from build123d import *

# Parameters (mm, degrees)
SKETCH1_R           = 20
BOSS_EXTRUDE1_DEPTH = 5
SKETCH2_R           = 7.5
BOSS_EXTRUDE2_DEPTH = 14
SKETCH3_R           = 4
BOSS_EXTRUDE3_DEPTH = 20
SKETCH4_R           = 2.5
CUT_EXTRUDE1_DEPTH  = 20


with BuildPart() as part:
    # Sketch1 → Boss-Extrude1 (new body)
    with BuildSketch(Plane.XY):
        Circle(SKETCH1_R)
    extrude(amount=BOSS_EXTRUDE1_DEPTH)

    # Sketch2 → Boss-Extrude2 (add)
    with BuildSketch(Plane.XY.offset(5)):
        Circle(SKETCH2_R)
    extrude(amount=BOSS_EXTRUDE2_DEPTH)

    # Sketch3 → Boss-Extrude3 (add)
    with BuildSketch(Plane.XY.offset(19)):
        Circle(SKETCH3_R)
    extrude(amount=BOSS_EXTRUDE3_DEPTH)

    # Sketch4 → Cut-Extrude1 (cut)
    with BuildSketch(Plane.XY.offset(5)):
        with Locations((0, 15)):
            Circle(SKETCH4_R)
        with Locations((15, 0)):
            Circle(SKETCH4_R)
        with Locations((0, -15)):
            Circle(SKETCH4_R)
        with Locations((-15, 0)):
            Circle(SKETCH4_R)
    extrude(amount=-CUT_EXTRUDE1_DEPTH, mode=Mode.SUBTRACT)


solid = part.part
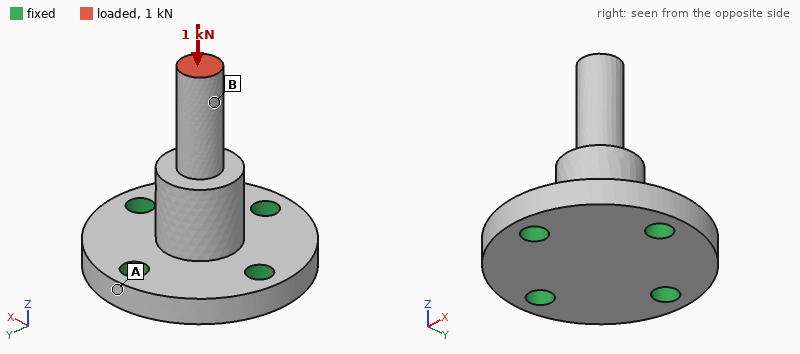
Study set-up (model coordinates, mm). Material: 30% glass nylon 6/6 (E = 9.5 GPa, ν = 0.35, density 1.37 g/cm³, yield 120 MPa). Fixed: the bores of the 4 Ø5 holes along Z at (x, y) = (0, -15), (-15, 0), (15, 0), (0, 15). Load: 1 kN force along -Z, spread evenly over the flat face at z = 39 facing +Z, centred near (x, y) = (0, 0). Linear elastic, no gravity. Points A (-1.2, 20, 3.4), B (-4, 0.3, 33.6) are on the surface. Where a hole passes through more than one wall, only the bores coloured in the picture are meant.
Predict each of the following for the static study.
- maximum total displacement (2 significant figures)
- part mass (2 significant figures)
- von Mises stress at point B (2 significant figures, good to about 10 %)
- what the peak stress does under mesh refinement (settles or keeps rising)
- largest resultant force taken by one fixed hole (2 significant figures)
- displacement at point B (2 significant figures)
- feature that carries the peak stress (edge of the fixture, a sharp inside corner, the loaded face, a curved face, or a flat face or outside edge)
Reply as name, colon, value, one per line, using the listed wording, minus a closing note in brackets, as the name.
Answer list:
maximum total displacement: 72 µm
part mass: 13 g
von Mises stress at point B: 20 MPa
what the peak stress does under mesh refinement: keeps rising
largest resultant force taken by one fixed hole: 260 N
displacement at point B: 61 µm
feature that carries the peak stress: edge of the fixture
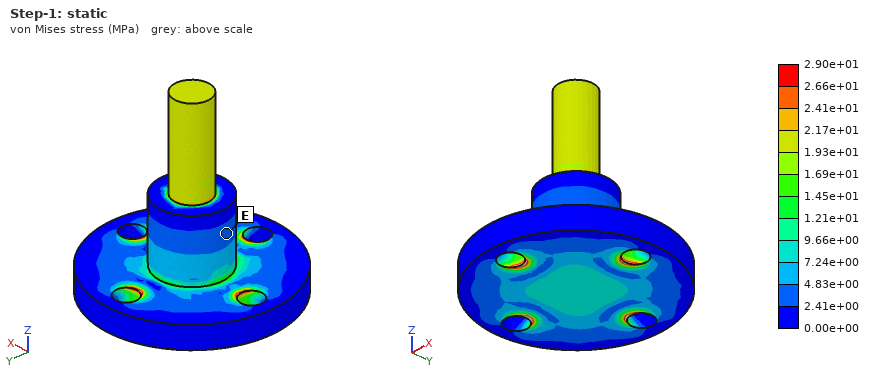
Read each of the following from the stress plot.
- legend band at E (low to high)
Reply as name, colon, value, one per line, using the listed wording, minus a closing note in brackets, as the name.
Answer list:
legend band at E: 2.41e+00 to 4.83e+00 MPa
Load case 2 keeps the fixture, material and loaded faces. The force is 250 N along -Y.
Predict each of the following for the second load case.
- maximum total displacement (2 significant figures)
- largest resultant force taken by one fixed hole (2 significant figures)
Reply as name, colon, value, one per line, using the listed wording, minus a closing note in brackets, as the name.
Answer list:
maximum total displacement: 0.68 mm
largest resultant force taken by one fixed hole: 370 N
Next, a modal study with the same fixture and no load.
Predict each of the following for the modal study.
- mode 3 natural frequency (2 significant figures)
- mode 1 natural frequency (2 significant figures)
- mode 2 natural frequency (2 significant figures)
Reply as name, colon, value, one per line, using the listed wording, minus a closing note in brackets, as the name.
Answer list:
mode 3 natural frequency: 12 kHz
mode 1 natural frequency: 4400 Hz
mode 2 natural frequency: 4400 Hz
